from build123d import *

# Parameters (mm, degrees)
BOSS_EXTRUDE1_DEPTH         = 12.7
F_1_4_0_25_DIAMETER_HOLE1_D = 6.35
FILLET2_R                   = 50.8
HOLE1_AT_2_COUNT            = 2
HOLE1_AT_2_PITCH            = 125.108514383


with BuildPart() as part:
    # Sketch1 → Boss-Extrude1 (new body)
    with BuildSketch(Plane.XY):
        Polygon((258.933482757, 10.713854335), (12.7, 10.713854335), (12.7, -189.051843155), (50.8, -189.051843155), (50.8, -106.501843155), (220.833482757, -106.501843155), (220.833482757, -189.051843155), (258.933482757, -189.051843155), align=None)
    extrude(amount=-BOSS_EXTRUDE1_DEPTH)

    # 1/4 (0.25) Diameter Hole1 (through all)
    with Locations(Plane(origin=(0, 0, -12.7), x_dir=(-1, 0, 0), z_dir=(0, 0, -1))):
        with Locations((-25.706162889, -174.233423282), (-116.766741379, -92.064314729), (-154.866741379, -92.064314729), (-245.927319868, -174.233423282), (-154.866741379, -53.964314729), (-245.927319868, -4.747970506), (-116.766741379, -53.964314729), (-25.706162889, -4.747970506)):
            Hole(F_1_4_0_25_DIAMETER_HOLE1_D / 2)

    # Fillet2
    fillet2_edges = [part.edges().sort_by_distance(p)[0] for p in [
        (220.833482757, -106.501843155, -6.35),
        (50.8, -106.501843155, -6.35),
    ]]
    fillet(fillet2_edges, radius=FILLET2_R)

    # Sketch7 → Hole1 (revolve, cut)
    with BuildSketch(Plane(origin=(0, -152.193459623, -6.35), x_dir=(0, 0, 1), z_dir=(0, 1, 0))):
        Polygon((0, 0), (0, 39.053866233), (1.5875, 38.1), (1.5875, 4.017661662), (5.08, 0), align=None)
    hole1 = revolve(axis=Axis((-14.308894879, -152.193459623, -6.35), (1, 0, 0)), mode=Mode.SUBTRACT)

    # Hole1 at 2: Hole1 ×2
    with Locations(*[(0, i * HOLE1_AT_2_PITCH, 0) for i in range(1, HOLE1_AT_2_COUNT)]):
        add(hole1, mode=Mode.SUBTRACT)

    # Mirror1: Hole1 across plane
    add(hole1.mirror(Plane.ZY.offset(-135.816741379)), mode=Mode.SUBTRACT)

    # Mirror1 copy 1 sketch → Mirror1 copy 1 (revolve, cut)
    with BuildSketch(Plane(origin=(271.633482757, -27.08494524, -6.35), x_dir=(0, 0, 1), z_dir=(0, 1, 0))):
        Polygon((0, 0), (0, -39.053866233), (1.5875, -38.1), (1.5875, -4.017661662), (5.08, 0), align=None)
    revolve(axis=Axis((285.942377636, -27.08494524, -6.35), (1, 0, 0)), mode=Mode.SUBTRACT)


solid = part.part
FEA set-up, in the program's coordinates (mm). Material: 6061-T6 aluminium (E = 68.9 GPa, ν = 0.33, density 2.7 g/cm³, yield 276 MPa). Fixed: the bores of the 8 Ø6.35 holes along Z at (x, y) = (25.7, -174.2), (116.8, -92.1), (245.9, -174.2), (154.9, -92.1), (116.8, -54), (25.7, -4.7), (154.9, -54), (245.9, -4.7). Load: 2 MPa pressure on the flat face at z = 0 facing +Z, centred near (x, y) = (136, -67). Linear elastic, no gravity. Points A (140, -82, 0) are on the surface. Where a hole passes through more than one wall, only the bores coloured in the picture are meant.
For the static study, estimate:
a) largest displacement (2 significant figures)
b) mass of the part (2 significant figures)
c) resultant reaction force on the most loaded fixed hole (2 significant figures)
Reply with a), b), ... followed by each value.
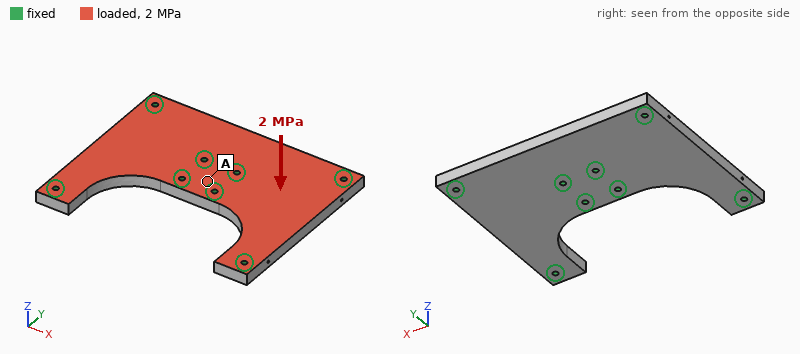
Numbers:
a) 0.40 mm
b) 1.2 kg
c) 12 kN
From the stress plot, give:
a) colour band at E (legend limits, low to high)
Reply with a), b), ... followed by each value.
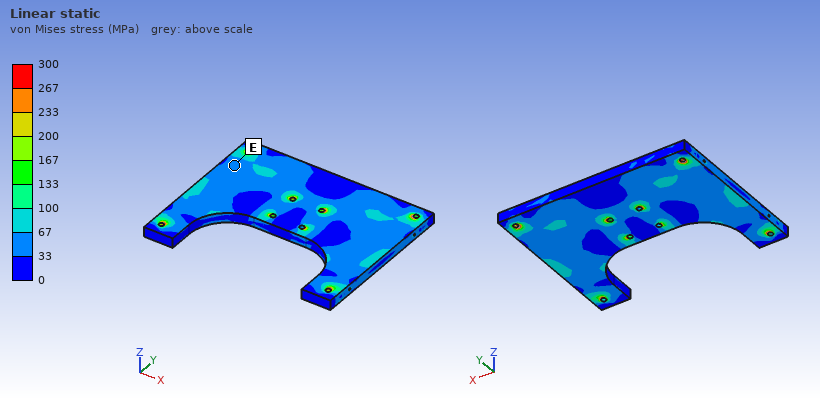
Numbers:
a) 33 to 67 MPa
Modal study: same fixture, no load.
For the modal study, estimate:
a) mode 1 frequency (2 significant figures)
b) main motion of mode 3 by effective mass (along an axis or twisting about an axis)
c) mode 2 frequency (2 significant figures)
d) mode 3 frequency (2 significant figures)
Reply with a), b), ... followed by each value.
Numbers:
a) 2400 Hz
b) along Z
c) 2400 Hz
d) 3000 Hz
